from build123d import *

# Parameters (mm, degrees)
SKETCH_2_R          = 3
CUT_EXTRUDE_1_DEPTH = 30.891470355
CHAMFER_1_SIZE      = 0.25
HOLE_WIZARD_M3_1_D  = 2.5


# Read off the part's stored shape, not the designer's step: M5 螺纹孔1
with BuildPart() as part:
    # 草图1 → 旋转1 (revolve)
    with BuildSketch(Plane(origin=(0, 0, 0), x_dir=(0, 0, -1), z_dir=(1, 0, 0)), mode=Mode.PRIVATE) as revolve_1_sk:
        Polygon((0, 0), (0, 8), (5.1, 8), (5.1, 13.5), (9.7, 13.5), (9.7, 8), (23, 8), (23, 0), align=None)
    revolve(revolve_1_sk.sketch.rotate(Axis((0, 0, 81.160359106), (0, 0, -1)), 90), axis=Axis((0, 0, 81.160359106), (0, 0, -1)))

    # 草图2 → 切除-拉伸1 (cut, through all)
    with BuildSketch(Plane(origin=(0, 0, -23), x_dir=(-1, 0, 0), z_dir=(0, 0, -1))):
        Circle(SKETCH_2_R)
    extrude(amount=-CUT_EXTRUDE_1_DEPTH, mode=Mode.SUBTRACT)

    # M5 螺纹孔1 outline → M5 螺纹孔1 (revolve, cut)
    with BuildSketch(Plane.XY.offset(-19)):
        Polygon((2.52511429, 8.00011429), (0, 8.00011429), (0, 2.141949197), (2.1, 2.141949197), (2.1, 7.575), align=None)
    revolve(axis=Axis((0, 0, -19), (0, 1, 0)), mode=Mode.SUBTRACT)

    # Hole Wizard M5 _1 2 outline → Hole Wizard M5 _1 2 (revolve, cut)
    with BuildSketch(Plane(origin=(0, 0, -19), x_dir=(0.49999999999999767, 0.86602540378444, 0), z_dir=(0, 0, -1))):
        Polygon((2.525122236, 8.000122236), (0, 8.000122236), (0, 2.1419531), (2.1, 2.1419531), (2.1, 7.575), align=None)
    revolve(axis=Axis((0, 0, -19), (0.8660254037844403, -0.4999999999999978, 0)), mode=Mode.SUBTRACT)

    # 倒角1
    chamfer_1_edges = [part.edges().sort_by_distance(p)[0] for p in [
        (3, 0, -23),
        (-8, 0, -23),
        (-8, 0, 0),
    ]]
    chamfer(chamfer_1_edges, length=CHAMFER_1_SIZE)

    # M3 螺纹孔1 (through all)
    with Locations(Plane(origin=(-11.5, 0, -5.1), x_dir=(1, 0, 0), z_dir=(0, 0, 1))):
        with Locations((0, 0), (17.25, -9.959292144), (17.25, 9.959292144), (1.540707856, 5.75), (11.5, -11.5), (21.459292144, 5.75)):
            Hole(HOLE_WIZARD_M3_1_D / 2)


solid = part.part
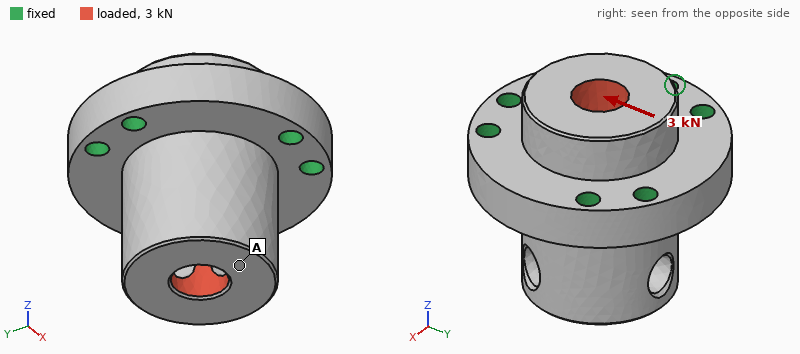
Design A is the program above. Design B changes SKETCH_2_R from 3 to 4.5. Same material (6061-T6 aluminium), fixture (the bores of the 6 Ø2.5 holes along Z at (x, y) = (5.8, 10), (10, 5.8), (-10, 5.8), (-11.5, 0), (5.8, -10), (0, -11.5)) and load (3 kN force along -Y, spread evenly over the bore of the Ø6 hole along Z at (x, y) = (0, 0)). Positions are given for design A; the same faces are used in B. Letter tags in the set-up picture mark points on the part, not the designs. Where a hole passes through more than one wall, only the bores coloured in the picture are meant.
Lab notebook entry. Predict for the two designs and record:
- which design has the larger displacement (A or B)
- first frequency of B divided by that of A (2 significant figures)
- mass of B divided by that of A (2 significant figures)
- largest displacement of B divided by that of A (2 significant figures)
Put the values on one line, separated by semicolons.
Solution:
B; 1.0; 0.86; 1.2
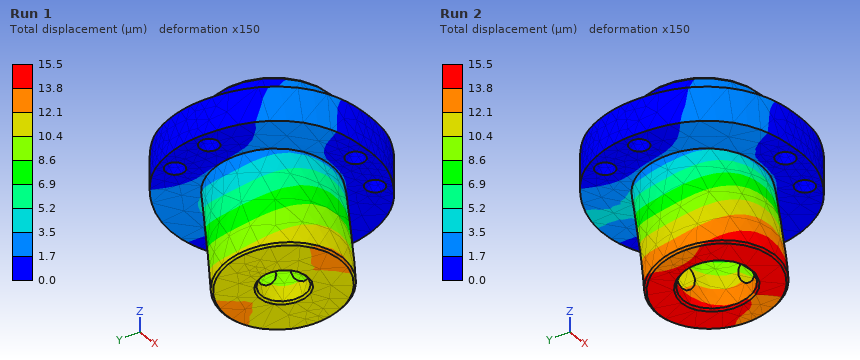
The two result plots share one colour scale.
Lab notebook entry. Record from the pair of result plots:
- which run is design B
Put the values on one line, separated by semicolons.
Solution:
Run 2
